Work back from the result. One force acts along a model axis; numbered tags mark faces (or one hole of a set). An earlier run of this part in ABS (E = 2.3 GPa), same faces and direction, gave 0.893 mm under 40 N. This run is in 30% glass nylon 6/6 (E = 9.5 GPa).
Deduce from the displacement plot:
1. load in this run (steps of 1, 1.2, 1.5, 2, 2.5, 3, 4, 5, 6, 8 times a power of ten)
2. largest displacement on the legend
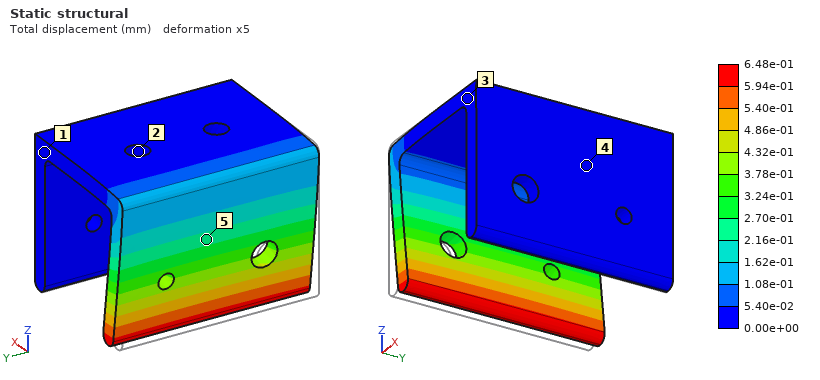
120 N
6.48e-01 mm
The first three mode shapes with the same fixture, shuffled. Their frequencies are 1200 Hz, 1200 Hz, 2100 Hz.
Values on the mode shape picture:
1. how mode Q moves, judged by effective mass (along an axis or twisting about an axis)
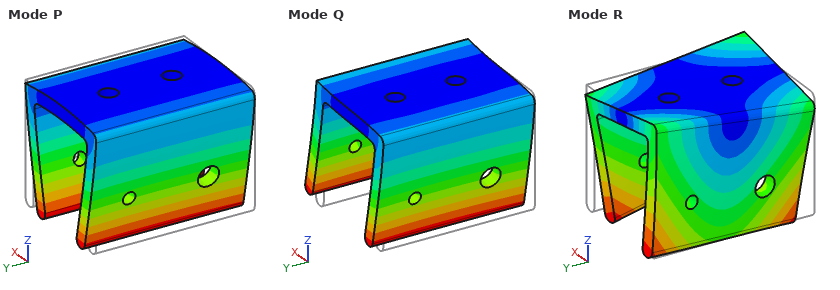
along X
